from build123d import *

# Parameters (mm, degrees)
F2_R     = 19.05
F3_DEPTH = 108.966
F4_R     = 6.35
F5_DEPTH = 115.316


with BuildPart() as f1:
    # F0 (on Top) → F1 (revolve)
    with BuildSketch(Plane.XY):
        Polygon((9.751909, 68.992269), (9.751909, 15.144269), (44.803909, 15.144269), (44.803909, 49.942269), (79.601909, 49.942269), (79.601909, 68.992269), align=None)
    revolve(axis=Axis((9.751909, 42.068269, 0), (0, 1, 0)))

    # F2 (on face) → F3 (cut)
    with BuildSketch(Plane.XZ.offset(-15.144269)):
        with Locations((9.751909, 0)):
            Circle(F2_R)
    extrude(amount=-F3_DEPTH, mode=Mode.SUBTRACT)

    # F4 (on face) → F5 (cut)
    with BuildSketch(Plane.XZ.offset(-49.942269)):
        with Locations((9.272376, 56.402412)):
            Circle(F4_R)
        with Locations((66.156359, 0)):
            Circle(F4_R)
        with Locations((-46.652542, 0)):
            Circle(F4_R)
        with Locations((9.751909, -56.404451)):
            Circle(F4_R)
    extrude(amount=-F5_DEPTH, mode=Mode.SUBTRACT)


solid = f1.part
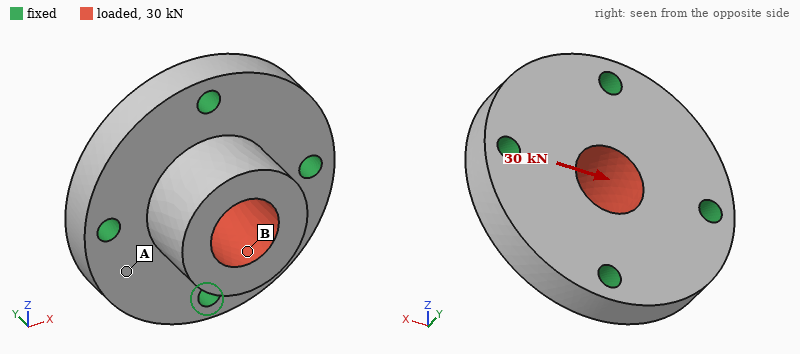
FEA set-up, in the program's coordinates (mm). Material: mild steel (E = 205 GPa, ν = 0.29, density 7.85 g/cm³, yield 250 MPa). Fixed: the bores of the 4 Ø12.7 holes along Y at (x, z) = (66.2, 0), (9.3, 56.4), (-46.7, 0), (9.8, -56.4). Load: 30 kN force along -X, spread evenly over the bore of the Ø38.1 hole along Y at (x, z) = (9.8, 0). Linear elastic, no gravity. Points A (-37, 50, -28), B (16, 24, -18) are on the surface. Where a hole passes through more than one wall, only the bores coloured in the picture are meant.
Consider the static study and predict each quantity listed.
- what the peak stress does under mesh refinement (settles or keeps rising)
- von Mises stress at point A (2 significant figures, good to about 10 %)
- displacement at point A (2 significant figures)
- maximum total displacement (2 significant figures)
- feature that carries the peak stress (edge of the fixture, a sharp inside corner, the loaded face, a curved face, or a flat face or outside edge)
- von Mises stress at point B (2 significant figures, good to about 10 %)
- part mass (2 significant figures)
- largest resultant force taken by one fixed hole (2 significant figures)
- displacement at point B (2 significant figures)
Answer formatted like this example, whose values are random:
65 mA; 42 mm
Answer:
keeps rising; 5.1 MPa; 1.9 µm; 9.7 µm; edge of the fixture; 14 MPa; 2.8 kg; 11 kN; 7.5 µm
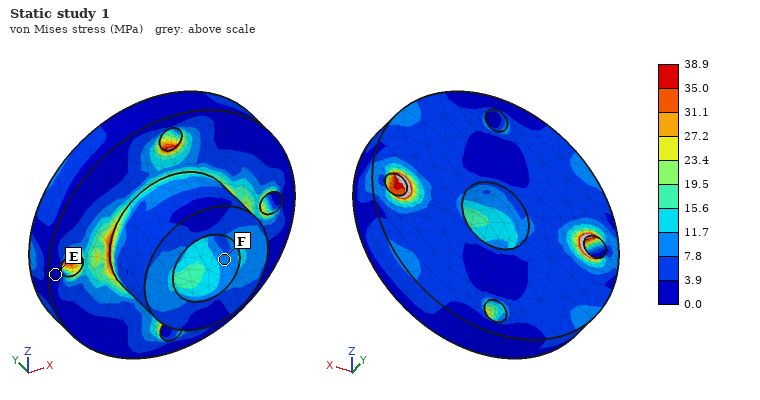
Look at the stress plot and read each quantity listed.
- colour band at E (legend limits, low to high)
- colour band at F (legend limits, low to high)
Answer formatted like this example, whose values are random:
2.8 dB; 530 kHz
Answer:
0.0 to 3.9 MPa; 7.8 to 11.7 MPa
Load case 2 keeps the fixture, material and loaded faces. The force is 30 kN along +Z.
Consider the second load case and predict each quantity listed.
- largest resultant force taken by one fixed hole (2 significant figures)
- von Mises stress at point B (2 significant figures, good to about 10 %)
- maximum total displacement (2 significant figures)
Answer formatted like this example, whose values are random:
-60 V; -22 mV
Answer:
11 kN; 8.9 MPa; 9.7 µm
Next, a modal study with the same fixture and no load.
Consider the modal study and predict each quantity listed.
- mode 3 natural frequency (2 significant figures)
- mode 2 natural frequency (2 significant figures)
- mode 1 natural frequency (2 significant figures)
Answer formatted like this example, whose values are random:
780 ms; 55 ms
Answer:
8800 Hz; 8700 Hz; 8700 Hz
